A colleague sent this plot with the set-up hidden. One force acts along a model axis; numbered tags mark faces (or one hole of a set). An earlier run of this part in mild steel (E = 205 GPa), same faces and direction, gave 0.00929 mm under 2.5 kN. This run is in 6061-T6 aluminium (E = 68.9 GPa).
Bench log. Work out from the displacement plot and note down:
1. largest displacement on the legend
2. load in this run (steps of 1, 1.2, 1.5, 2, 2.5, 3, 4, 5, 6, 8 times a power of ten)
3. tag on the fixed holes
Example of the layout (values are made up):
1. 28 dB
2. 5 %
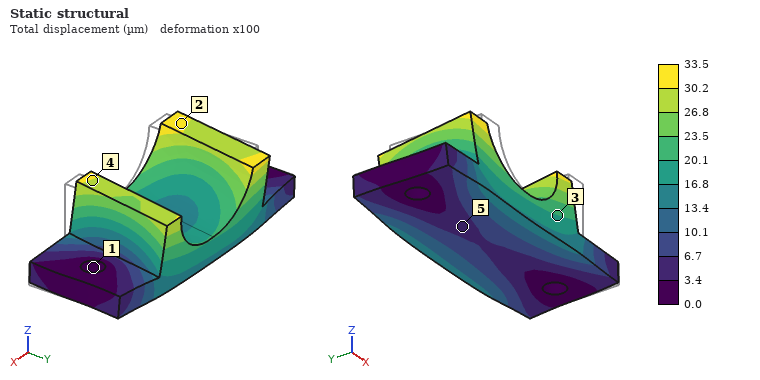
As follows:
1. 33.5 µm
2. 3 kN
3. 1
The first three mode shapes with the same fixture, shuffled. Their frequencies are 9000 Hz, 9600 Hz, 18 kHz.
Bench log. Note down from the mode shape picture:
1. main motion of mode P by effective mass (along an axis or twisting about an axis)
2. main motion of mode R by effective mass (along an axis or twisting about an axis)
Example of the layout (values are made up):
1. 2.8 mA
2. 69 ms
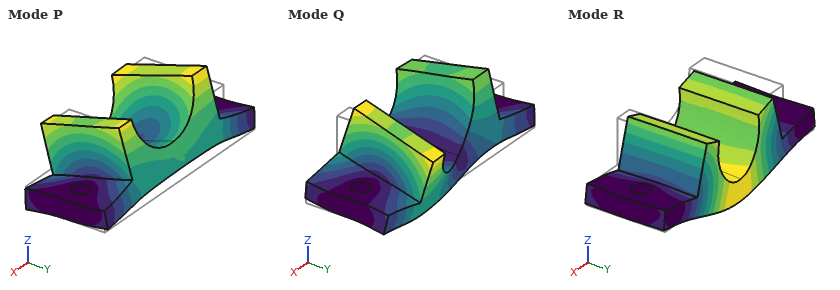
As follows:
1. along Y
2. along Z
